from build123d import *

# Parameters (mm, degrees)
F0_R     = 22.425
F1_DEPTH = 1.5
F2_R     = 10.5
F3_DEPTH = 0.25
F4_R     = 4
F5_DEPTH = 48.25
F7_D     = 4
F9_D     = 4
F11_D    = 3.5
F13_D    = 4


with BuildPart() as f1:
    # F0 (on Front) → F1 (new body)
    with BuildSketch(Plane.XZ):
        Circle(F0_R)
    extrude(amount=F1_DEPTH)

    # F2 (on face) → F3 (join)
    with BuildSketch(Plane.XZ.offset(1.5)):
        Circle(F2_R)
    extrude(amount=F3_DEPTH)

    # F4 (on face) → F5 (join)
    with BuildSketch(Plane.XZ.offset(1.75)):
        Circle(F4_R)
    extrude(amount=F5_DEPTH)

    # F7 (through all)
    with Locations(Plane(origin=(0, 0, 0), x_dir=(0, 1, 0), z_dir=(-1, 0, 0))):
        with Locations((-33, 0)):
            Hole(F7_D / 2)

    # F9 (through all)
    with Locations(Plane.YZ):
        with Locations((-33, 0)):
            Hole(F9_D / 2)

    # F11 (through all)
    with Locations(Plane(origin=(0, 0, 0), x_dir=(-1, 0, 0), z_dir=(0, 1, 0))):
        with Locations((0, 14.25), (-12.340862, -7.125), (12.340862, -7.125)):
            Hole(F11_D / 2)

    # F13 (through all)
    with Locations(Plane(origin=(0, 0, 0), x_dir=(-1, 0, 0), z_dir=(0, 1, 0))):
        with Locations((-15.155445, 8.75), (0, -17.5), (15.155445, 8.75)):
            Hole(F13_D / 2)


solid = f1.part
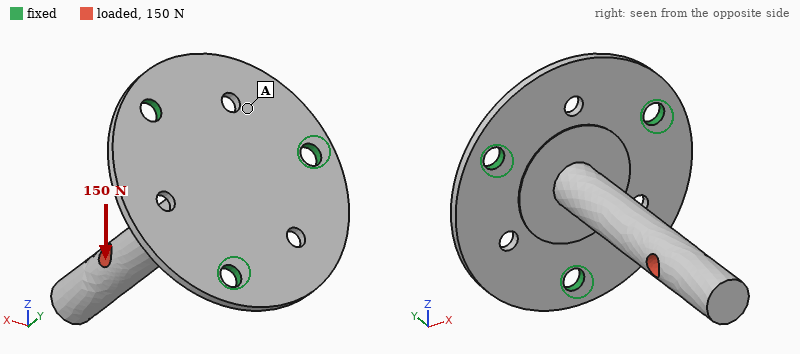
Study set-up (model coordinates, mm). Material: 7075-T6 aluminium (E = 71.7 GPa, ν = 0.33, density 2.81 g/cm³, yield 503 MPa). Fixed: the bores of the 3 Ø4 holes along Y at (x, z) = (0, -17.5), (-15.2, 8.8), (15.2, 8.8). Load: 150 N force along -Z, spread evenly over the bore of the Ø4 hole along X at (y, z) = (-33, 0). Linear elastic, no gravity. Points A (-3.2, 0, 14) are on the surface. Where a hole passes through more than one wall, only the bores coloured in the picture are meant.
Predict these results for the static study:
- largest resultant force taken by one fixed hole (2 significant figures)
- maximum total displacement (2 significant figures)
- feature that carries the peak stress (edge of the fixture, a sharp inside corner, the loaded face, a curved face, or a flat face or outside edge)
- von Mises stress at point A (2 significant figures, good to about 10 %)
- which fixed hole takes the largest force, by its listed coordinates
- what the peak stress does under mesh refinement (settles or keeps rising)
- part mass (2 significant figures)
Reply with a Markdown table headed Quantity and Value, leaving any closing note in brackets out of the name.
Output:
| Quantity | Value |
|---|---|
| largest resultant force taken by one fixed hole | 230 N |
| maximum total displacement | 0.75 mm |
| feature that carries the peak stress | edge of the fixture |
| von Mises stress at point A | 30 MPa |
| which fixed hole takes the largest force, by its listed coordinates | (0, -17.5) |
| what the peak stress does under mesh refinement | keeps rising |
| part mass | 13 g |
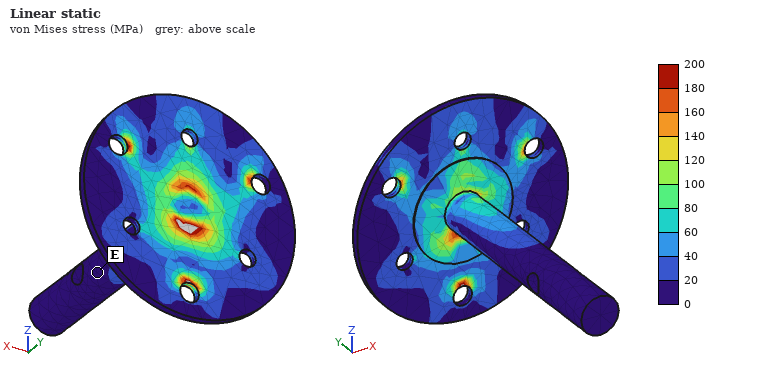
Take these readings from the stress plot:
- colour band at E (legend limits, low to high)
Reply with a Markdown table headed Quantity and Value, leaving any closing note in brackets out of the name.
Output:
| Quantity | Value |
|---|---|
| colour band at E | 0 to 20 MPa |
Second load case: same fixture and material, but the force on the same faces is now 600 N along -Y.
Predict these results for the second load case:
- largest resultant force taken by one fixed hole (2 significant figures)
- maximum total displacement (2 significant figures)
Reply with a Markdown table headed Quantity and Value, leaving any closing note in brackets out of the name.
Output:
| Quantity | Value |
|---|---|
| largest resultant force taken by one fixed hole | 240 N |
| maximum total displacement | 0.10 mm |
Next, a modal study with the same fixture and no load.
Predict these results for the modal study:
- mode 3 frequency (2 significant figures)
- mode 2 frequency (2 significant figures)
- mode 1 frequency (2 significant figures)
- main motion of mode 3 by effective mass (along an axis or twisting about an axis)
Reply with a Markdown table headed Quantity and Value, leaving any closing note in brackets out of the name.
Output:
| Quantity | Value |
|---|---|
| mode 3 frequency | 4400 Hz |
| mode 2 frequency | 1200 Hz |
| mode 1 frequency | 1200 Hz |
| main motion of mode 3 by effective mass | along Y |
